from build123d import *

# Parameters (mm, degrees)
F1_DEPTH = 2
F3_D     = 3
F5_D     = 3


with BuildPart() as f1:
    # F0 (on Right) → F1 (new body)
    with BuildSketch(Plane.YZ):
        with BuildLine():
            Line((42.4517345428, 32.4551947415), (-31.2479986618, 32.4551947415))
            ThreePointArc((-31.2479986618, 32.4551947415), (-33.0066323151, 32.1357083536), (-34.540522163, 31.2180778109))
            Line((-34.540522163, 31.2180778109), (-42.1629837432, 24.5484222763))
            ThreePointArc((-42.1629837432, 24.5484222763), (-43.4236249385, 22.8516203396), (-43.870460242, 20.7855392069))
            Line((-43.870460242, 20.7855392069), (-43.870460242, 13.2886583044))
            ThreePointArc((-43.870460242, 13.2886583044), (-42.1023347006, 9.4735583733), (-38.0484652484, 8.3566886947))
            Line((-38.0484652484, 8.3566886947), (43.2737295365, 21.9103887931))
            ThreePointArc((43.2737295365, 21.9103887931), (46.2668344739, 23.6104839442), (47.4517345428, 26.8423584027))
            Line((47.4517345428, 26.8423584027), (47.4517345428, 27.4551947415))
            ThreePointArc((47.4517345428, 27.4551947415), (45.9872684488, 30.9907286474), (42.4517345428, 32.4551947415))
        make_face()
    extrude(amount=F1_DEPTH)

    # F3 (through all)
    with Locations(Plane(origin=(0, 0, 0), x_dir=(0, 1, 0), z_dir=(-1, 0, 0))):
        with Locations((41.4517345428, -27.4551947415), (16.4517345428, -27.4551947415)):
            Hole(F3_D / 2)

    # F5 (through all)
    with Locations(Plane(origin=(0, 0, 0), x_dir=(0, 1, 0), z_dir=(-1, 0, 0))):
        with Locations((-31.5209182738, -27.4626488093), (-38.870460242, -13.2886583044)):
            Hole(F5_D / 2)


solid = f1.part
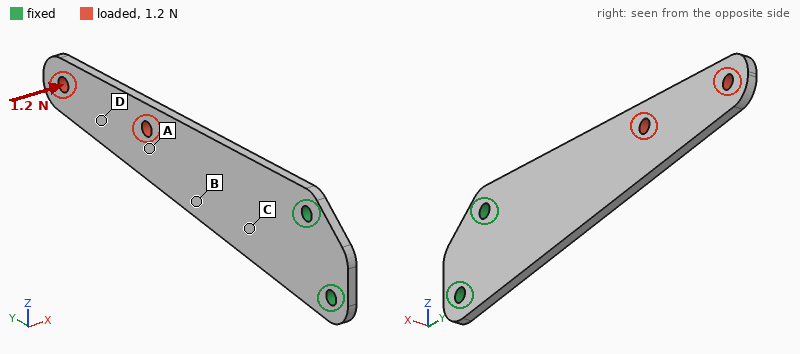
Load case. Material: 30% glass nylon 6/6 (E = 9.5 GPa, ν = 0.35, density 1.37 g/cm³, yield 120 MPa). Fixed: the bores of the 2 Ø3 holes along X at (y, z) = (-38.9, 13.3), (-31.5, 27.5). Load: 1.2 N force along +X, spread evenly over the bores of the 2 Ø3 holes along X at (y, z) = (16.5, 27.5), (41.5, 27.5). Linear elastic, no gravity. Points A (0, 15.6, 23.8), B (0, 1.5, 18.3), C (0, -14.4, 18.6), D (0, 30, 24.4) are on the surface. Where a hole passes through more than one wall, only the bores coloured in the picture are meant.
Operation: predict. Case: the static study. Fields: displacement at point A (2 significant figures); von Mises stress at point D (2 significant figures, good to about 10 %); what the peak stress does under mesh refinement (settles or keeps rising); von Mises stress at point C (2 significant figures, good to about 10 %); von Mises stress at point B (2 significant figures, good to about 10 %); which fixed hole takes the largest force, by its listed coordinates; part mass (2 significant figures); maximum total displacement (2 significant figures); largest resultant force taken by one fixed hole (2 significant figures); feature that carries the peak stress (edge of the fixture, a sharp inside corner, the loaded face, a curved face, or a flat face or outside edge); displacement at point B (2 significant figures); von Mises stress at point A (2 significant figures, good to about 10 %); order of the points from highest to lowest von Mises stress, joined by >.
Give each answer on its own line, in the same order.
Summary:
0.47 mm
0.85 MPa
keeps rising
3.8 MPa
2.9 MPa
(-31.5, 27.5)
4.1 g
1.1 mm
3.1 N
edge of the fixture
0.25 mm
1.9 MPa
C > B > A > D
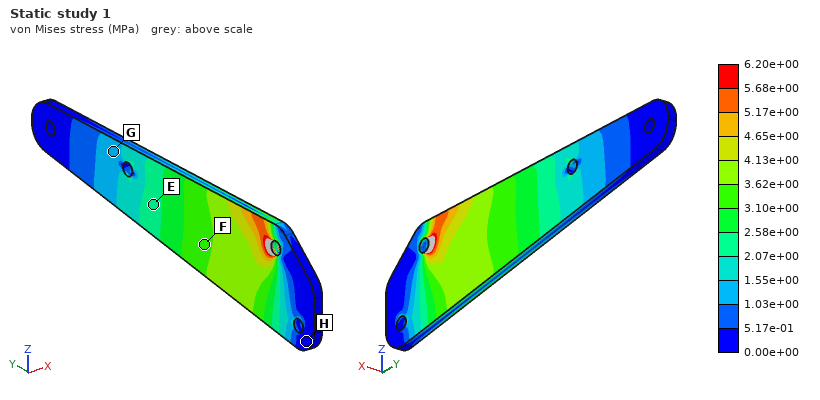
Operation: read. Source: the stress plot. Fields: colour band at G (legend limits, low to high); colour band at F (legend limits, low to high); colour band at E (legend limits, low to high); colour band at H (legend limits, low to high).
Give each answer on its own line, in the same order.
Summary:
1.03e+00 to 1.55e+00 MPa
3.10e+00 to 3.62e+00 MPa
2.07e+00 to 2.58e+00 MPa
0.00e+00 to 5.17e-01 MPa
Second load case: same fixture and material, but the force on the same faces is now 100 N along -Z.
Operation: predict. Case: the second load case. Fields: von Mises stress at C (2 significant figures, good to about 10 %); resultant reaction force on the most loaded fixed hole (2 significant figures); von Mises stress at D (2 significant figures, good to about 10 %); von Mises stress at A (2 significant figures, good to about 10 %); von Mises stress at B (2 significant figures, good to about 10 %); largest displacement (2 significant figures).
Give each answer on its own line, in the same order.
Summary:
13 MPa
390 N
5.0 MPa
6.7 MPa
18 MPa
1.1 mm
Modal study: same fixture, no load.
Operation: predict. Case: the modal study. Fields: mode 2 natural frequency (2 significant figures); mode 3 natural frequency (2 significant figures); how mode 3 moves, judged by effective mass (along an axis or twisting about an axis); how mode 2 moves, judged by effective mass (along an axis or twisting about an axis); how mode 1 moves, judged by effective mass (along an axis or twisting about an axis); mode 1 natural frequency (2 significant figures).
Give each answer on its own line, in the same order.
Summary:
920 Hz
1600 Hz
along Z
along X
along X
180 Hz
